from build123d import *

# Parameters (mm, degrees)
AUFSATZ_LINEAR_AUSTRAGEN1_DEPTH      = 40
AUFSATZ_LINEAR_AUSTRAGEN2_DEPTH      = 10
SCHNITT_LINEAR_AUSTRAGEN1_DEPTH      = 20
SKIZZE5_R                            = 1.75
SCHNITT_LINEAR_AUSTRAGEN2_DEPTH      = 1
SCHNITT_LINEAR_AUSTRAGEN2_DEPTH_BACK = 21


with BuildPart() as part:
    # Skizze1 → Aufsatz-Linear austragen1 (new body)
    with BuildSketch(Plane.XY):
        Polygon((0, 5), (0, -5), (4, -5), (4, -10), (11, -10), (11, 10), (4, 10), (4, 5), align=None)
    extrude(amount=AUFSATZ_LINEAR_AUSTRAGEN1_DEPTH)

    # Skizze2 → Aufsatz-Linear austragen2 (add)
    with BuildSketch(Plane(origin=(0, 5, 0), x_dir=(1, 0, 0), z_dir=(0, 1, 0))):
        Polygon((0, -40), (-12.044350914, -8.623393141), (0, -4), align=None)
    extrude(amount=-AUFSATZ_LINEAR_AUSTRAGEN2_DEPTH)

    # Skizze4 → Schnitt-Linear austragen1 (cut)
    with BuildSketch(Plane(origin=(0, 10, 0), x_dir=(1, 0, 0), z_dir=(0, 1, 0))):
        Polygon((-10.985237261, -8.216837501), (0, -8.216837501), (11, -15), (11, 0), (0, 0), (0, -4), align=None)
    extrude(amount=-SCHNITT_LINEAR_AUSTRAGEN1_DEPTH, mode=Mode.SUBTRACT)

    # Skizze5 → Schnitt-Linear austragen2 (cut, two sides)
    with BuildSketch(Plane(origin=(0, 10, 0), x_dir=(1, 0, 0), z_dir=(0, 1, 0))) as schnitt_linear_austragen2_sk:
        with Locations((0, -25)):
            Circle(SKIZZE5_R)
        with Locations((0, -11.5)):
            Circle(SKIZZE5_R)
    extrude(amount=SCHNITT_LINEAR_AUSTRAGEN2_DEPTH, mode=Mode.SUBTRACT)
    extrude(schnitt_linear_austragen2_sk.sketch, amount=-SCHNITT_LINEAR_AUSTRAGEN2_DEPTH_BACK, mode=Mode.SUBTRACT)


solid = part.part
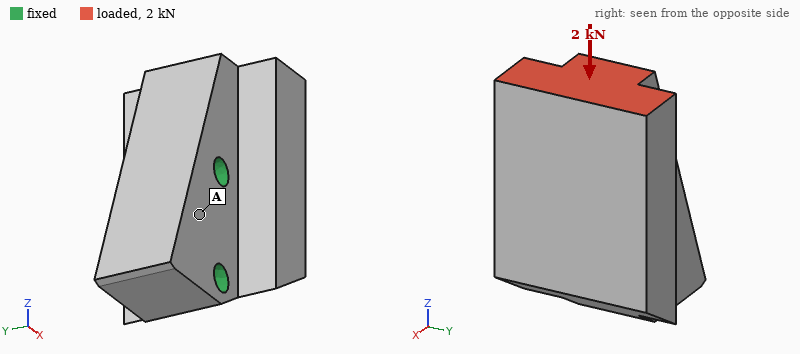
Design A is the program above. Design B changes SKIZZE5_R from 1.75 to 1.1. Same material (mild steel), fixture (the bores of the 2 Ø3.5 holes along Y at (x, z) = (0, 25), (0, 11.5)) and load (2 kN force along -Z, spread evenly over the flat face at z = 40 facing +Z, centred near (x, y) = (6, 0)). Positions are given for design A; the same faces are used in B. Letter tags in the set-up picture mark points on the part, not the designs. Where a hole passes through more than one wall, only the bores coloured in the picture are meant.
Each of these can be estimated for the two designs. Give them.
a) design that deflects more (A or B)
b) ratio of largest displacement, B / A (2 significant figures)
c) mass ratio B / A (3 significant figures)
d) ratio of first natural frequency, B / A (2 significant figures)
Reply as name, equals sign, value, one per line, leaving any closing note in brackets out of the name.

design that deflects more = B
ratio of largest displacement, B / A = 1.2
mass ratio B / A = 1.02
ratio of first natural frequency, B / A = 0.89
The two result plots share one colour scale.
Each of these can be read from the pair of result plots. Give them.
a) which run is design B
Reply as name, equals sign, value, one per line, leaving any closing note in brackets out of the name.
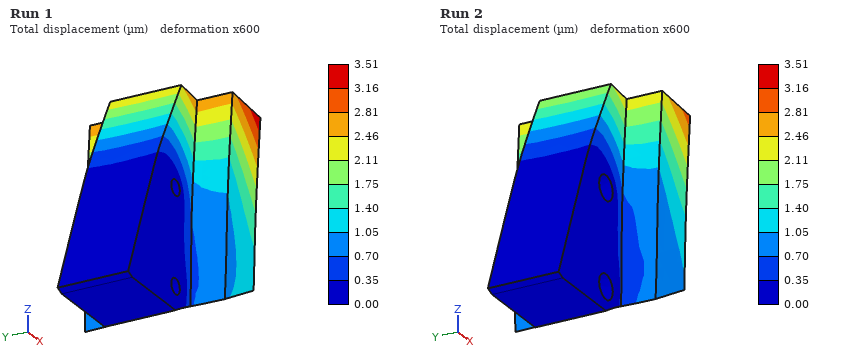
which run is design B = Run 1
